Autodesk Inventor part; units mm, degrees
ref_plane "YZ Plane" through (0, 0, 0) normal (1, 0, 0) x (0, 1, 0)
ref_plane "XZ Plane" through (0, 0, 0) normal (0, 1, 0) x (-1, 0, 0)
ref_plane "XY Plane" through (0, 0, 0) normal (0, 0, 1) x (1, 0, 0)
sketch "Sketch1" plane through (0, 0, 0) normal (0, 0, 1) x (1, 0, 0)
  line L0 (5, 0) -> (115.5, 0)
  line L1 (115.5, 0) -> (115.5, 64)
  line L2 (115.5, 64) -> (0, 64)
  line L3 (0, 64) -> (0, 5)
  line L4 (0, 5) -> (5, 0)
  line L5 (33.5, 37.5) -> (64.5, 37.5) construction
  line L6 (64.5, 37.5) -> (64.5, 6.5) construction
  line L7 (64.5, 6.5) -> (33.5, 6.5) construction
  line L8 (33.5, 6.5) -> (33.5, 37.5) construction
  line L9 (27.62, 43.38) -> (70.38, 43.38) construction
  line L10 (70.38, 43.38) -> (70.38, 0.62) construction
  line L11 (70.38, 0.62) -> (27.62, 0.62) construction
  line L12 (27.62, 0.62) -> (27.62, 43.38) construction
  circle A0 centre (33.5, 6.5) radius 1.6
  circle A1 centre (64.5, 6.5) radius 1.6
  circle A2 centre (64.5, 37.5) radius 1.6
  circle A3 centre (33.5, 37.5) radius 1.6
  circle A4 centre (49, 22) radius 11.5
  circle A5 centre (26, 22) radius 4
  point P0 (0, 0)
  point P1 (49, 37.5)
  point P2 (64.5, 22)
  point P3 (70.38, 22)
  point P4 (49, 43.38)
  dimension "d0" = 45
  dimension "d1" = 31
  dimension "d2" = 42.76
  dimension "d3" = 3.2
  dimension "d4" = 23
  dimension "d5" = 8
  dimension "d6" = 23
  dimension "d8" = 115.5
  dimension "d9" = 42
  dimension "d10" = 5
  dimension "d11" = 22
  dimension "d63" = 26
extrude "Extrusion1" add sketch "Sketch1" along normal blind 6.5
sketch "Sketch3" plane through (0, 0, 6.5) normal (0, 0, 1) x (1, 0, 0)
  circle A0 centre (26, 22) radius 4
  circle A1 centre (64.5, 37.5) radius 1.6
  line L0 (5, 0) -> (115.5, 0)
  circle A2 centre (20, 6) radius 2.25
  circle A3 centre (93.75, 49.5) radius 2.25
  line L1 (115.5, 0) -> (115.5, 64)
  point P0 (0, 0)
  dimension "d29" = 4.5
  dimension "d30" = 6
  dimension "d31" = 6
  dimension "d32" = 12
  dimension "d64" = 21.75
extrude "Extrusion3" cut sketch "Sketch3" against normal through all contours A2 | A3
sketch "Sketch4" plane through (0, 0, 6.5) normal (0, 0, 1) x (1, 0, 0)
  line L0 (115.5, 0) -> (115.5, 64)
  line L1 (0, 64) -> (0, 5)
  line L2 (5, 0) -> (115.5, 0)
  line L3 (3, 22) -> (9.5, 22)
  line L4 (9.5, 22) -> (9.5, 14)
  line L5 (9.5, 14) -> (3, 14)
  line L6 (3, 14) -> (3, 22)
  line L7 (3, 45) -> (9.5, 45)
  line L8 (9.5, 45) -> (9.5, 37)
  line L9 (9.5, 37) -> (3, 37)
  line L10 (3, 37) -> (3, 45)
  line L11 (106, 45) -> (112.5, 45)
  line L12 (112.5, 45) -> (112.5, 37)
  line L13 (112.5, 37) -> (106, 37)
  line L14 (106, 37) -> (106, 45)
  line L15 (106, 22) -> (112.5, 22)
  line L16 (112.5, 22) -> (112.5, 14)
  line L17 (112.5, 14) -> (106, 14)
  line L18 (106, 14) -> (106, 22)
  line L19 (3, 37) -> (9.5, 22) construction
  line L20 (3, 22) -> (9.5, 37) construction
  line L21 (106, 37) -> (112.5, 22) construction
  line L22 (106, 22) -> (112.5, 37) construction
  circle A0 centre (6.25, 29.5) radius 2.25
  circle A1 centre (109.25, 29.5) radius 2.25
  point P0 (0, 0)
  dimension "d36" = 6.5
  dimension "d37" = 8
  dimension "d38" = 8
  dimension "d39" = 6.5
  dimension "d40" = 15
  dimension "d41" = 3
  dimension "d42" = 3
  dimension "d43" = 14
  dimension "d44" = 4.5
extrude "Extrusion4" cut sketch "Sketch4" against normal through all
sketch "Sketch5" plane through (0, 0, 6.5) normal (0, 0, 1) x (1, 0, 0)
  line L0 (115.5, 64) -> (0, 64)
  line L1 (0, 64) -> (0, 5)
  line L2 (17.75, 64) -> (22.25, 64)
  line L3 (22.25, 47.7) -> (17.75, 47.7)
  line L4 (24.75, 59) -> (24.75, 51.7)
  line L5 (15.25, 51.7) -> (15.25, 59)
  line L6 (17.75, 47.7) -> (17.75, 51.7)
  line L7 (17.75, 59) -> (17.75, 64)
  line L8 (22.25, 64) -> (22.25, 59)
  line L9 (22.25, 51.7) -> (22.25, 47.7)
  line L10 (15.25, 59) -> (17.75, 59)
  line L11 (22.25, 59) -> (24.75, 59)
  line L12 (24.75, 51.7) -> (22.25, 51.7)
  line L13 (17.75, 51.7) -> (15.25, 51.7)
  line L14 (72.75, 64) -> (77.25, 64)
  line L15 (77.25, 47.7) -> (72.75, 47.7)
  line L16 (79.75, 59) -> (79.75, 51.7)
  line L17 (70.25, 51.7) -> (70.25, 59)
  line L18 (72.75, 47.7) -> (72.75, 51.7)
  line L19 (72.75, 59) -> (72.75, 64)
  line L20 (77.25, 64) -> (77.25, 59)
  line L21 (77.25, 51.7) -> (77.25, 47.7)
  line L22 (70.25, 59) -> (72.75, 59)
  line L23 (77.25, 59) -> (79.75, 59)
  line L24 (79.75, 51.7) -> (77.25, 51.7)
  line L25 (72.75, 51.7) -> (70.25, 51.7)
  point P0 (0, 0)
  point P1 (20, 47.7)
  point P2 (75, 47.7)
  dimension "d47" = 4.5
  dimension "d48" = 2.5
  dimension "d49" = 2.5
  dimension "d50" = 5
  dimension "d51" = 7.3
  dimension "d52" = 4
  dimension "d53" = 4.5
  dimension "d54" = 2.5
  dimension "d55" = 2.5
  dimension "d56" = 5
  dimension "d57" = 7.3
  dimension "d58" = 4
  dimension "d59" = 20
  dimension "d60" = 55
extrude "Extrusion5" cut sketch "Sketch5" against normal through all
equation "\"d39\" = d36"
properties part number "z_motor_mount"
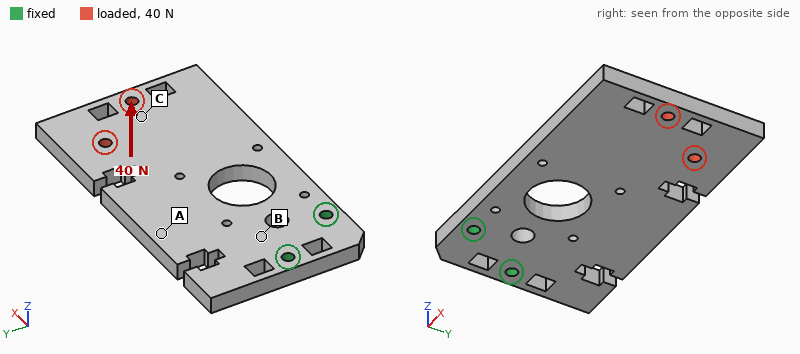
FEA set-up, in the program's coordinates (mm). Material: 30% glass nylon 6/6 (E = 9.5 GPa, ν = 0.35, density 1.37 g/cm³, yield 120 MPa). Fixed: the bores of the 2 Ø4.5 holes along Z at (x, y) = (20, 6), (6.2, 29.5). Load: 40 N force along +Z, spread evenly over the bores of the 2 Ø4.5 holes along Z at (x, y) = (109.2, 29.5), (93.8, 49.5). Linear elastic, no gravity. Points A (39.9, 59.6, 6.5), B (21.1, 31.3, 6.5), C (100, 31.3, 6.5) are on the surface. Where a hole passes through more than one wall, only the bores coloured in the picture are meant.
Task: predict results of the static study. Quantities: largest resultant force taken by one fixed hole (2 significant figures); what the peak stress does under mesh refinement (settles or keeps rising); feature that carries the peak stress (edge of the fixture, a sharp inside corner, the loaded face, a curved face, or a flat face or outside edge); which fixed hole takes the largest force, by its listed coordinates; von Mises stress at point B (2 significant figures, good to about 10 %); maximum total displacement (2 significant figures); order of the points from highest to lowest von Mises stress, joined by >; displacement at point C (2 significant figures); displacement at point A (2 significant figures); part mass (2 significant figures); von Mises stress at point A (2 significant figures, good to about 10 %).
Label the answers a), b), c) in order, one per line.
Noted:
a) 48 N
b) keeps rising
c) edge of the fixture
d) (20, 6)
e) 9.3 MPa
f) 1.5 mm
g) B > A > C
h) 1.1 mm
i) 0.26 mm
j) 57 g
k) 4.7 MPa
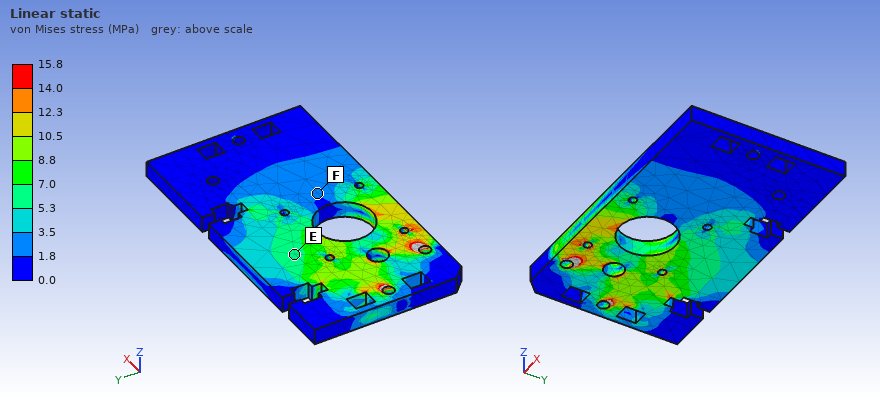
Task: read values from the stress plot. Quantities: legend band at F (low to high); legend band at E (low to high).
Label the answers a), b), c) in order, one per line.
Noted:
a) 1.8 to 3.5 MPa
b) 5.3 to 7.0 MPa
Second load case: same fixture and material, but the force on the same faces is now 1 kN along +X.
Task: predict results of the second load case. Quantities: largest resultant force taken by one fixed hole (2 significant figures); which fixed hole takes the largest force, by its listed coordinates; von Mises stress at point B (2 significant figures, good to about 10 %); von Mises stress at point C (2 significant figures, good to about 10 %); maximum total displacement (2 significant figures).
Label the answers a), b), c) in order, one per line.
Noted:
a) 1.2 kN
b) (6.2, 29.5)
c) 9.0 MPa
d) 5.2 MPa
e) 0.25 mm
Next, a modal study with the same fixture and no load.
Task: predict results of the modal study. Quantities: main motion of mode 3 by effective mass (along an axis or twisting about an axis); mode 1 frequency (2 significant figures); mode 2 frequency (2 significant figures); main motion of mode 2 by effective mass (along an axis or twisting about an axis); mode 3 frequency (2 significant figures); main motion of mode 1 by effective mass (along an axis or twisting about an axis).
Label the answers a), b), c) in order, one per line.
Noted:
a) along Y
b) 210 Hz
c) 680 Hz
d) twisting about X
e) 1100 Hz
f) along Z
